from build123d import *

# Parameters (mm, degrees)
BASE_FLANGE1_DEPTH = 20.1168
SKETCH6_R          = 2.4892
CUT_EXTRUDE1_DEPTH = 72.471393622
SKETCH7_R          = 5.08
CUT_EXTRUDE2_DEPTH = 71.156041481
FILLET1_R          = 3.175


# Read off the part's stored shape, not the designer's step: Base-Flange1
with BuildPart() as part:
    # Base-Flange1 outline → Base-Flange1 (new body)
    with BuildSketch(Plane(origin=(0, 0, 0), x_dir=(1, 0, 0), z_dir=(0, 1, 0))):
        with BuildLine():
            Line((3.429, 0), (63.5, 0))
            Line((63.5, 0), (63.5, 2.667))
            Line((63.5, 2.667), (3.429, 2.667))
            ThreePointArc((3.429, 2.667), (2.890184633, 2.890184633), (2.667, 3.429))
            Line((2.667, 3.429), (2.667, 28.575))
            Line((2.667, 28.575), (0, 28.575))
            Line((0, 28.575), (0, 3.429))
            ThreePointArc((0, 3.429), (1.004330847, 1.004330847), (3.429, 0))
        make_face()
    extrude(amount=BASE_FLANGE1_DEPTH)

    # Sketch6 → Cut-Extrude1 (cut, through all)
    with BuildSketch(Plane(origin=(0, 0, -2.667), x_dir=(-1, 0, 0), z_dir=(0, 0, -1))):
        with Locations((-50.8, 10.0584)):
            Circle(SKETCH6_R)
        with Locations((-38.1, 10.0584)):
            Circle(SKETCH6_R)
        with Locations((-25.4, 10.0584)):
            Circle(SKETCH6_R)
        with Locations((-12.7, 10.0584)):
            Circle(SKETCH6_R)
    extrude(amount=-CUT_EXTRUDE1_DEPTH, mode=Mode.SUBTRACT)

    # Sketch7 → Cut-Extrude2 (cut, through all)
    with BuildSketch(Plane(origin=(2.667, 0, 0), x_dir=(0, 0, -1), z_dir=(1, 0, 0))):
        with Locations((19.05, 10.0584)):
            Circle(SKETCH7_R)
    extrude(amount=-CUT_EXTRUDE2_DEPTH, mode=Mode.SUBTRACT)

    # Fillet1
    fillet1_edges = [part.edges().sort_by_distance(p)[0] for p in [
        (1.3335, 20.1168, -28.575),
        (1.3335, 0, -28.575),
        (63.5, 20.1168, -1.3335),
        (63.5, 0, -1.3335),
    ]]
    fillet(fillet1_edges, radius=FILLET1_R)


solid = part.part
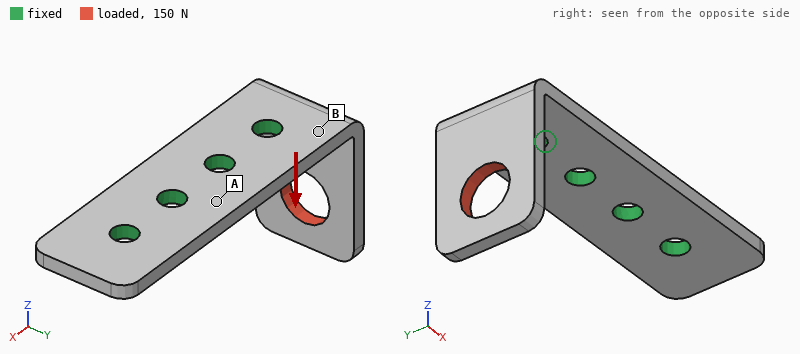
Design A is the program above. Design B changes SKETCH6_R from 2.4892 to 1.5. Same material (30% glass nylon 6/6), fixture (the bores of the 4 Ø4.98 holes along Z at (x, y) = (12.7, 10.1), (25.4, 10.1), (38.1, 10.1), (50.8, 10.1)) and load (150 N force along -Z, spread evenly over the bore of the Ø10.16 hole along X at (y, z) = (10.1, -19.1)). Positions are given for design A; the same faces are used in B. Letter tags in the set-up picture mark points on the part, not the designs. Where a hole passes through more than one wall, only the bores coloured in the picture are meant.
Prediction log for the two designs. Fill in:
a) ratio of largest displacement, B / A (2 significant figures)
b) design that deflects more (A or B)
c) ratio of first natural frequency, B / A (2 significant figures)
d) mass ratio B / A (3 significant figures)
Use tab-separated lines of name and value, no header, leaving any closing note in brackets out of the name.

ratio of largest displacement, B / A	1.3
design that deflects more	B
ratio of first natural frequency, B / A	0.95
mass ratio B / A	1.03
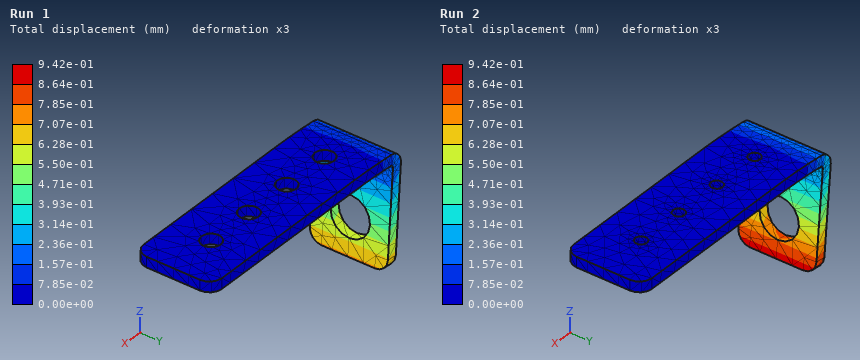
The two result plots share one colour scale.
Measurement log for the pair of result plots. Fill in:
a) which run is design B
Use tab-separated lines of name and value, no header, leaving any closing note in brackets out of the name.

which run is design B	Run 2
